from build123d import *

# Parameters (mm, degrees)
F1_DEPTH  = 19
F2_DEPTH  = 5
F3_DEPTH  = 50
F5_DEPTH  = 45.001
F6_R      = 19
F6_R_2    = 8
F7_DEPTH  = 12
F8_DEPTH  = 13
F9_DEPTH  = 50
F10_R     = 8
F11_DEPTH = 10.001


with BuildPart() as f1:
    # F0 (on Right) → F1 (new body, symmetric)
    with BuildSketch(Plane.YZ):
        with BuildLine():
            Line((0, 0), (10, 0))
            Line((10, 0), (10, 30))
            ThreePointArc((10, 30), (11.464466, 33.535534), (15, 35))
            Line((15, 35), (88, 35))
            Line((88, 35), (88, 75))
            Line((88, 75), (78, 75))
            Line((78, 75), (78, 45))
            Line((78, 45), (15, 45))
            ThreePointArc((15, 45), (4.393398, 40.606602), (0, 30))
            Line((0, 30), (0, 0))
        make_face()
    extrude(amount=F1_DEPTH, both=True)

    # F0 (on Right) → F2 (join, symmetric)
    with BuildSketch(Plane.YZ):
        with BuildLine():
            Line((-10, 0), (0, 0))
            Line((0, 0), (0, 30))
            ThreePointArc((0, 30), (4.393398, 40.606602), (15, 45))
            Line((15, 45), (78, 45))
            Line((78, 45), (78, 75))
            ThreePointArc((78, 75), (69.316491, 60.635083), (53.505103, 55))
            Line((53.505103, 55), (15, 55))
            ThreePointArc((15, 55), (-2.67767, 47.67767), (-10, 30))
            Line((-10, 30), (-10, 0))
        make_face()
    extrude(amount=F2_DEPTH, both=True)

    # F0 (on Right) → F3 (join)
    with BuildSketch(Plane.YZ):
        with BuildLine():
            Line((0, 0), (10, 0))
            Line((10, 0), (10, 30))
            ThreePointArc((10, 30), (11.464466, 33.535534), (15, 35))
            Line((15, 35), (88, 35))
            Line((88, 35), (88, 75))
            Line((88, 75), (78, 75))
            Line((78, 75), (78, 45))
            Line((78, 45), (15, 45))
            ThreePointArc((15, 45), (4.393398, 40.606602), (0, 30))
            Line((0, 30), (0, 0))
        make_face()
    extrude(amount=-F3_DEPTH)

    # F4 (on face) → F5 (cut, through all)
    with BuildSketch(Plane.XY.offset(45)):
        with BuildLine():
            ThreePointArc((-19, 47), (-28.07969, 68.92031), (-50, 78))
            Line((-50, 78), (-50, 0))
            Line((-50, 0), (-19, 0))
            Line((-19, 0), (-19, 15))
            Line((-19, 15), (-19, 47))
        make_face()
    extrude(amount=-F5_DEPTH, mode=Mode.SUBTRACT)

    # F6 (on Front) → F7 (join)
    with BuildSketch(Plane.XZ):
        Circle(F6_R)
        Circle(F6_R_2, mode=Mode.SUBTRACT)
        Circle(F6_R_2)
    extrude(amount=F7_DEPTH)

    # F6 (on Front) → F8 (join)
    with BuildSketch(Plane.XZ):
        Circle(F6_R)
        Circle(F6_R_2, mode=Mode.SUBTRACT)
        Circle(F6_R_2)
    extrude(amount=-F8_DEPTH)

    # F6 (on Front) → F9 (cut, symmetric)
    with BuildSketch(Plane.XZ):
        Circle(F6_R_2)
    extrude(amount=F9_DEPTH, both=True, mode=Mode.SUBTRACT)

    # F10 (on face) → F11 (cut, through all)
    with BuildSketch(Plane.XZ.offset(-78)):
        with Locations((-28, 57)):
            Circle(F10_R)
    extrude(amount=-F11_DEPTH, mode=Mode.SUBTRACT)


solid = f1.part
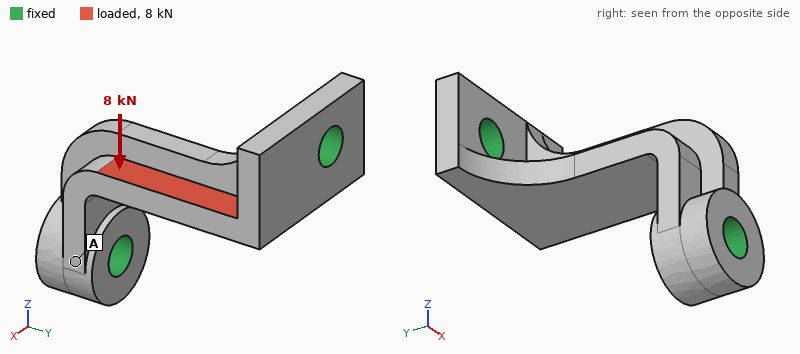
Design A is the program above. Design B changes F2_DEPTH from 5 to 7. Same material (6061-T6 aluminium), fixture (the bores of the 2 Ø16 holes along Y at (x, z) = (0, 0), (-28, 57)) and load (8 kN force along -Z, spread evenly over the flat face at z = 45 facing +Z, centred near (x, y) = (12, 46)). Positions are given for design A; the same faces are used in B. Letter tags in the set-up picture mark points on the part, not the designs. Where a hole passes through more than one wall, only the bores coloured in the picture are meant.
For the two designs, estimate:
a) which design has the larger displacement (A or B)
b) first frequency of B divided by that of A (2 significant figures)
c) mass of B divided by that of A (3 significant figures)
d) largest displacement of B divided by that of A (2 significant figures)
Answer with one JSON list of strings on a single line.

["A", "1.00", "1.05", "0.91"]
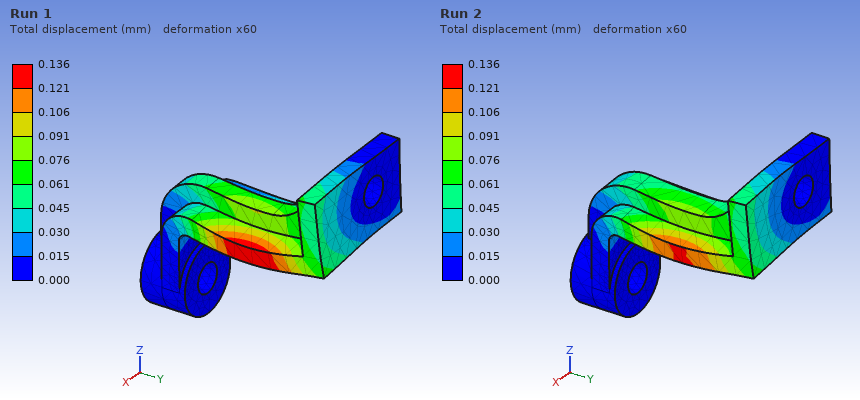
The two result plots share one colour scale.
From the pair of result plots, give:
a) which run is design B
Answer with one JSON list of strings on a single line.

["Run 2"]
